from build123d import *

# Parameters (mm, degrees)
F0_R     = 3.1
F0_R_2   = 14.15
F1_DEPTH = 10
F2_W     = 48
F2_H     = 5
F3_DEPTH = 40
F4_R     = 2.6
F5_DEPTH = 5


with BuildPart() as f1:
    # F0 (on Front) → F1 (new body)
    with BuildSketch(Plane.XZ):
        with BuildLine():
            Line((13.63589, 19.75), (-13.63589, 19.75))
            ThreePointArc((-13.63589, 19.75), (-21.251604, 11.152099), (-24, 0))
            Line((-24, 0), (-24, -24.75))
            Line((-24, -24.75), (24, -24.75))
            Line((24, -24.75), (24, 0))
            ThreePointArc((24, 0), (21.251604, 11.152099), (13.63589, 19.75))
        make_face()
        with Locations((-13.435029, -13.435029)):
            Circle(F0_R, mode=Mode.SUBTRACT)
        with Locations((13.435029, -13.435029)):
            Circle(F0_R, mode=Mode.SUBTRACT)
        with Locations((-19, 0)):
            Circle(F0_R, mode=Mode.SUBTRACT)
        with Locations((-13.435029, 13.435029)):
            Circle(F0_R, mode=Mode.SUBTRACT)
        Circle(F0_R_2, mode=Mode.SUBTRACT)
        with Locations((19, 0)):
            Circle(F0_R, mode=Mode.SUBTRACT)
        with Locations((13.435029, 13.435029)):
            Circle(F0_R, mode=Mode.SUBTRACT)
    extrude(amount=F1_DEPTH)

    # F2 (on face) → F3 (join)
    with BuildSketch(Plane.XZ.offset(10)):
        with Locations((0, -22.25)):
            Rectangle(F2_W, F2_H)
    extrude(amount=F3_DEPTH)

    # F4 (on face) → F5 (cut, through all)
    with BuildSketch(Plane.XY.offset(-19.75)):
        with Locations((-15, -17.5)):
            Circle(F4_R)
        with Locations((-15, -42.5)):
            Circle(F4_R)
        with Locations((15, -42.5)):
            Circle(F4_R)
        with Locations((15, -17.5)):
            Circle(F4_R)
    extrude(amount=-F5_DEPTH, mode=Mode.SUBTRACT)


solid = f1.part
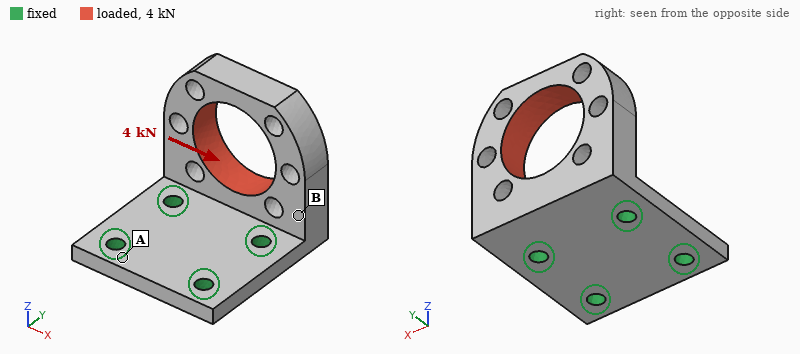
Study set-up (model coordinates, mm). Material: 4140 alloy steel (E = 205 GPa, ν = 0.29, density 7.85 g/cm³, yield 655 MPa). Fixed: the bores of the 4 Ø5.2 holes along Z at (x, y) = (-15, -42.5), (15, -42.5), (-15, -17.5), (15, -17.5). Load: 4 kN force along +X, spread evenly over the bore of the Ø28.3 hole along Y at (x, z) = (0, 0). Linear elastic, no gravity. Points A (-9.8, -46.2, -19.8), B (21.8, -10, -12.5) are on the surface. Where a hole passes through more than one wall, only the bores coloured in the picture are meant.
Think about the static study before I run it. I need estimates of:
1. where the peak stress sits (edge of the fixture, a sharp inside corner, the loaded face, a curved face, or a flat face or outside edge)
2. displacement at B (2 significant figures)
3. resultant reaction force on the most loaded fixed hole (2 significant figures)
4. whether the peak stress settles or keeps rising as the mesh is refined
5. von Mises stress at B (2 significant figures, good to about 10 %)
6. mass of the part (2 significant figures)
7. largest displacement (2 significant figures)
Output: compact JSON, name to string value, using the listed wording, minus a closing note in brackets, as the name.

{"where the peak stress sits": "edge of the fixture", "displacement at B": "25 µm", "resultant reaction force on the most loaded fixed hole": "3.5 kN", "whether the peak stress settles or keeps rising as the mesh is refined": "keeps rising", "von Mises stress at B": "59 MPa", "mass of the part": "170 g", "largest displacement": "75 µm"}
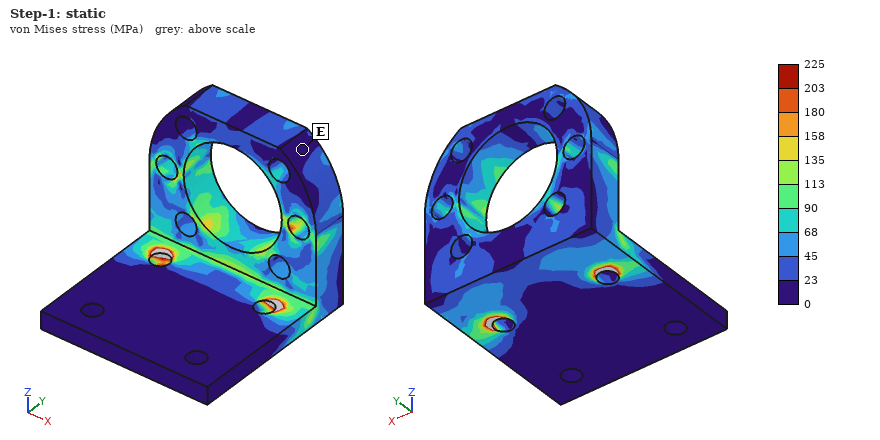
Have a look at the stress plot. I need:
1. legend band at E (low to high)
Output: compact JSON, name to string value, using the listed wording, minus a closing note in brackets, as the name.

{"legend band at E": "0 to 23 MPa"}
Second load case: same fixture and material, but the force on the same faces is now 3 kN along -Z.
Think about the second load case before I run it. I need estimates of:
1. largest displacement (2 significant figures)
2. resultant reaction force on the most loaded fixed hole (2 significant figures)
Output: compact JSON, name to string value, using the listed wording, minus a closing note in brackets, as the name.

{"largest displacement": "95 µm", "resultant reaction force on the most loaded fixed hole": "1.6 kN"}
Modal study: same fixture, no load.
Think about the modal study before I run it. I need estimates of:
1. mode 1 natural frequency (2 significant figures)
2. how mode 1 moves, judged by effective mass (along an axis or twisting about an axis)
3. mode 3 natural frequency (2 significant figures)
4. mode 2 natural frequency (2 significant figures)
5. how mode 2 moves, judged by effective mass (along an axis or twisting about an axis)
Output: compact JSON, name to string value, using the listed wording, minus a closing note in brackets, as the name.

{"mode 1 natural frequency": "2100 Hz", "how mode 1 moves, judged by effective mass": "along Y", "mode 3 natural frequency": "7100 Hz", "mode 2 natural frequency": "4700 Hz", "how mode 2 moves, judged by effective mass": "along X"}
